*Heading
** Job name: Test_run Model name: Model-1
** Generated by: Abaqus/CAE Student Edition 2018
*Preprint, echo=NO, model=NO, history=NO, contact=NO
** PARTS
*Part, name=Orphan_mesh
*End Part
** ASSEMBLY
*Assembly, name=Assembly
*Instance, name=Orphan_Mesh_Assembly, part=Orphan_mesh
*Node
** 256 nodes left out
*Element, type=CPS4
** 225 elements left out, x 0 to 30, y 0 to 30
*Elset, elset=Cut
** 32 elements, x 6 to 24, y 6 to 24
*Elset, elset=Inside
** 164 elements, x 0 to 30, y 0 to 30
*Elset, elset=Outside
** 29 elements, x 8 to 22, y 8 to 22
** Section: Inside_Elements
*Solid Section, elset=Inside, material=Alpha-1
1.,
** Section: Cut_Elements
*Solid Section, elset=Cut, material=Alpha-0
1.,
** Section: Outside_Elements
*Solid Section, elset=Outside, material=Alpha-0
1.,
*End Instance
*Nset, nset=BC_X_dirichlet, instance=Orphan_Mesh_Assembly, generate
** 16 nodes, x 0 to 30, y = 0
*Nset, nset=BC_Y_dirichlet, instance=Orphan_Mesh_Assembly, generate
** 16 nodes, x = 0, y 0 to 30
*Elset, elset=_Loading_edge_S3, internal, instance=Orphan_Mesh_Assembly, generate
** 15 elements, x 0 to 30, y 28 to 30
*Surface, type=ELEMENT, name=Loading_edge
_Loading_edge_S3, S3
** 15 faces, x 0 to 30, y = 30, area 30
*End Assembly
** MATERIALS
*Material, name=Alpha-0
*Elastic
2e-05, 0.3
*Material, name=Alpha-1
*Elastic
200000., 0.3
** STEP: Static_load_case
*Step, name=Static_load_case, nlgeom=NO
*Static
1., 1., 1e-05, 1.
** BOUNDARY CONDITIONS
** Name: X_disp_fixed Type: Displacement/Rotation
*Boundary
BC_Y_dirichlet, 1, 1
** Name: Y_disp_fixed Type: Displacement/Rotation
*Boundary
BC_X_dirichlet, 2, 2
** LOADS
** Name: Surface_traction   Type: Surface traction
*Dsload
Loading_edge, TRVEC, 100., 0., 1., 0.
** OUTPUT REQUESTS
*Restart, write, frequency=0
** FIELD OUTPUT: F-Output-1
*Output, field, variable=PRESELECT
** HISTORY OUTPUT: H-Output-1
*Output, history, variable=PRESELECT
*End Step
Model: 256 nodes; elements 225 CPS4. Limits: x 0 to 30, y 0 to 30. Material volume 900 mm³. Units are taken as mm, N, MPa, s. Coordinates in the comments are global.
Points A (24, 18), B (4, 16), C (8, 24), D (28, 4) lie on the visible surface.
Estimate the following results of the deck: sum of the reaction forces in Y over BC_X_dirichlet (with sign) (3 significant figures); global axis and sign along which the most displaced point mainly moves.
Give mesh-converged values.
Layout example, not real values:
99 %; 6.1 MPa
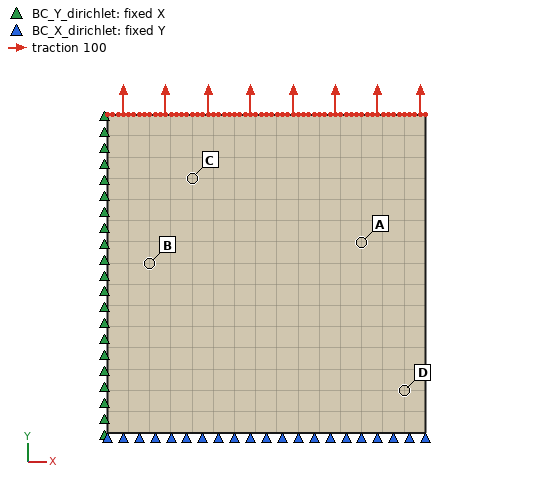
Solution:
-3000 N; +Y
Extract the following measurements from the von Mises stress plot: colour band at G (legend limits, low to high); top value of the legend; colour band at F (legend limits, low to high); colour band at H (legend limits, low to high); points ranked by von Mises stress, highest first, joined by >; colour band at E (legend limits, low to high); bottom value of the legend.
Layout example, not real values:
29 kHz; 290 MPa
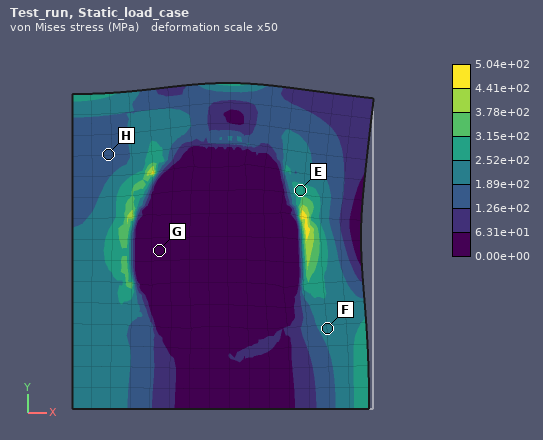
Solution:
0.00e+00 to 6.31e+01 MPa; 5.04e+02 MPa; 1.89e+02 to 2.52e+02 MPa; 1.26e+02 to 1.89e+02 MPa; E > F > H > G; 2.52e+02 to 3.15e+02 MPa; 0.00e+00 MPa
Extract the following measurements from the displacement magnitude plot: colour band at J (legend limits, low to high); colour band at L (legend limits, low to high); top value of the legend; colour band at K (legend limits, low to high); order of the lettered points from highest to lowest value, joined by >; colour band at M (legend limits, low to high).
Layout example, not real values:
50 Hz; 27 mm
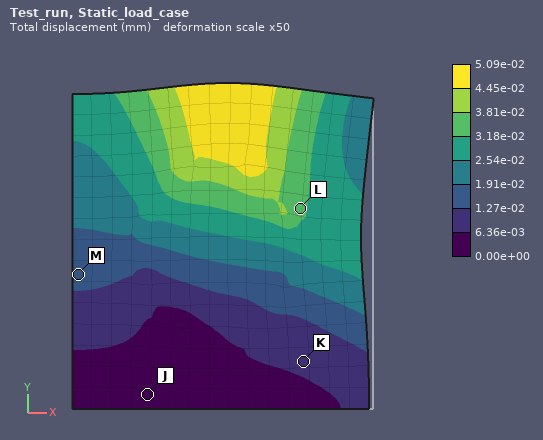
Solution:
0.00e+00 to 6.36e-03 mm; 3.18e-02 to 3.81e-02 mm; 5.09e-02 mm; 6.36e-03 to 1.27e-02 mm; L > M > K > J; 1.27e-02 to 1.91e-02 mm
